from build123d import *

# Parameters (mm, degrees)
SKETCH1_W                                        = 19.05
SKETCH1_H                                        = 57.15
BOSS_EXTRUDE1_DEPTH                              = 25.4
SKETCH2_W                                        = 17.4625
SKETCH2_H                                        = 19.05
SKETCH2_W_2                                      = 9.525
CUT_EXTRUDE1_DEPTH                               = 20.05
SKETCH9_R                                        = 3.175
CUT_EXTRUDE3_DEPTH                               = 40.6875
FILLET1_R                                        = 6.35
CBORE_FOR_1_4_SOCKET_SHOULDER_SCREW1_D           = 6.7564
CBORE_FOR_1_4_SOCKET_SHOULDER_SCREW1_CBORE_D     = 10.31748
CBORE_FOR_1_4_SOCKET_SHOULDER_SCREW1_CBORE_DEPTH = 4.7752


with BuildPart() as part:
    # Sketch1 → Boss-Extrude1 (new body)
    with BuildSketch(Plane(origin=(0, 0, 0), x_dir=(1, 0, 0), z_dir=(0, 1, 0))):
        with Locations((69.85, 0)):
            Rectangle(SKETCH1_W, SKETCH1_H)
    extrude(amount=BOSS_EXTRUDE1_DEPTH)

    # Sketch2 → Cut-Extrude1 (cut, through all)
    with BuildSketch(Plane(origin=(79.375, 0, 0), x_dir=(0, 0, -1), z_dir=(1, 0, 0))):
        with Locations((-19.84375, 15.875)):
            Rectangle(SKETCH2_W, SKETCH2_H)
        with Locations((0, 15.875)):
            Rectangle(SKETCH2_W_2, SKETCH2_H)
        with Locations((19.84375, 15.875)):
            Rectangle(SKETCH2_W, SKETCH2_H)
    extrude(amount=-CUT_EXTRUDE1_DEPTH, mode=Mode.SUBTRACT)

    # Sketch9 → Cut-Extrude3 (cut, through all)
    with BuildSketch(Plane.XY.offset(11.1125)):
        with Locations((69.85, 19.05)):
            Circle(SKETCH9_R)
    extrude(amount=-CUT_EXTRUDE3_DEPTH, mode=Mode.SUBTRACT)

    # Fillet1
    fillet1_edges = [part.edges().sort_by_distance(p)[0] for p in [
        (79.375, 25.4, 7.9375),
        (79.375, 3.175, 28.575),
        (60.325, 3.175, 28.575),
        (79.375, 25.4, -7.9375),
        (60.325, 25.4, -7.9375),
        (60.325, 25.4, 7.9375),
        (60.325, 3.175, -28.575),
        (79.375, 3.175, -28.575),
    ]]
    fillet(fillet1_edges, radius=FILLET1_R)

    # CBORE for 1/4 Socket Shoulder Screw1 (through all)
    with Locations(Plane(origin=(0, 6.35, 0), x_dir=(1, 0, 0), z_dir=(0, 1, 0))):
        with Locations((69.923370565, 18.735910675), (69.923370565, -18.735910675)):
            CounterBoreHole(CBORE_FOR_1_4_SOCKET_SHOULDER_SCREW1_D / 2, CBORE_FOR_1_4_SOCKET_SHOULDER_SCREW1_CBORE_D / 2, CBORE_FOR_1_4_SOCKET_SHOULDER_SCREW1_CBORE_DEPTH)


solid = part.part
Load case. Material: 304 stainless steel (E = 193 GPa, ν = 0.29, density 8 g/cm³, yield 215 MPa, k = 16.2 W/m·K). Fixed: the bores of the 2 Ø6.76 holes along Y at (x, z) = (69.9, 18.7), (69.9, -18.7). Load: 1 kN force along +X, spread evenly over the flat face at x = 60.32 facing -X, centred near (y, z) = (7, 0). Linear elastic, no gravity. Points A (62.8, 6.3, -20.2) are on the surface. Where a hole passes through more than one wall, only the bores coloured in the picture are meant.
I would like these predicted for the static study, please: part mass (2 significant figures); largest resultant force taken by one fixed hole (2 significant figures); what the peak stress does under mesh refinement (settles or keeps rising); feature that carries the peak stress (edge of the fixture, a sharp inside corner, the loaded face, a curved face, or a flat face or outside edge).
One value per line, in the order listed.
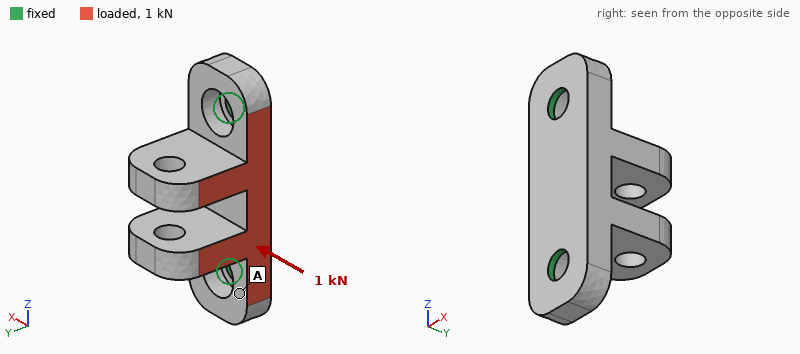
78 g
500 N
keeps rising
edge of the fixture
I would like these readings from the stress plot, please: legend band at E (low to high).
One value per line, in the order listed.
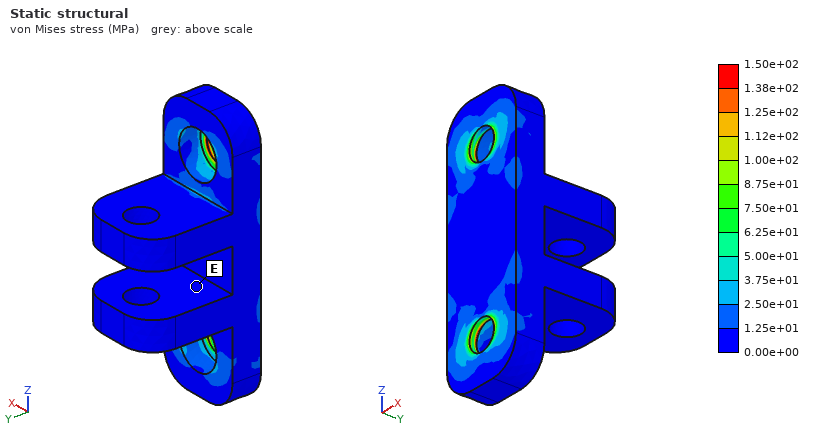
0.00e+00 to 1.25e+01 MPa
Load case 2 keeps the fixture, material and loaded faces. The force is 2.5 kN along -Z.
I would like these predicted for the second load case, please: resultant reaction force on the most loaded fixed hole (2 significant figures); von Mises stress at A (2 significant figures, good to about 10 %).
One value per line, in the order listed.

1.4 kN
13 MPa
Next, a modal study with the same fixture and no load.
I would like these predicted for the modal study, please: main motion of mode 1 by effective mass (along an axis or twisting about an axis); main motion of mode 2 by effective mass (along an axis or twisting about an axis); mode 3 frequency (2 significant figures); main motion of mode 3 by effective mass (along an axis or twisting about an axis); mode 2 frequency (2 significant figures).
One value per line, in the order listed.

along X
along Y
11 kHz
along Z
7800 Hz
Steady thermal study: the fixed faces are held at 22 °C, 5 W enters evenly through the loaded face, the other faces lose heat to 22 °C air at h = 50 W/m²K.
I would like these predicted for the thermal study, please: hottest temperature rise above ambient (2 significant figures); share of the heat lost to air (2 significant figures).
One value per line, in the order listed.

16 K
41 %
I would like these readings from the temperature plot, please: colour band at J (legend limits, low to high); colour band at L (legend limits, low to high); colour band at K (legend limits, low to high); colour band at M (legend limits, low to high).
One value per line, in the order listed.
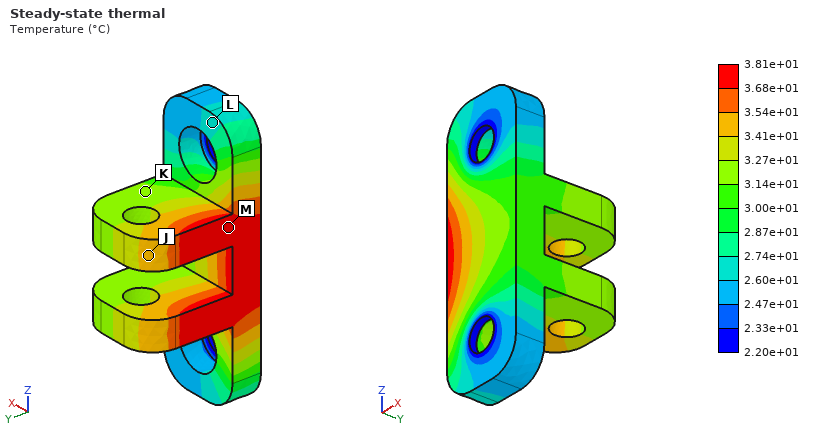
3.41e+01 to 3.54e+01 °C
2.60e+01 to 2.74e+01 °C
3.14e+01 to 3.27e+01 °C
3.68e+01 to 3.81e+01 °C
